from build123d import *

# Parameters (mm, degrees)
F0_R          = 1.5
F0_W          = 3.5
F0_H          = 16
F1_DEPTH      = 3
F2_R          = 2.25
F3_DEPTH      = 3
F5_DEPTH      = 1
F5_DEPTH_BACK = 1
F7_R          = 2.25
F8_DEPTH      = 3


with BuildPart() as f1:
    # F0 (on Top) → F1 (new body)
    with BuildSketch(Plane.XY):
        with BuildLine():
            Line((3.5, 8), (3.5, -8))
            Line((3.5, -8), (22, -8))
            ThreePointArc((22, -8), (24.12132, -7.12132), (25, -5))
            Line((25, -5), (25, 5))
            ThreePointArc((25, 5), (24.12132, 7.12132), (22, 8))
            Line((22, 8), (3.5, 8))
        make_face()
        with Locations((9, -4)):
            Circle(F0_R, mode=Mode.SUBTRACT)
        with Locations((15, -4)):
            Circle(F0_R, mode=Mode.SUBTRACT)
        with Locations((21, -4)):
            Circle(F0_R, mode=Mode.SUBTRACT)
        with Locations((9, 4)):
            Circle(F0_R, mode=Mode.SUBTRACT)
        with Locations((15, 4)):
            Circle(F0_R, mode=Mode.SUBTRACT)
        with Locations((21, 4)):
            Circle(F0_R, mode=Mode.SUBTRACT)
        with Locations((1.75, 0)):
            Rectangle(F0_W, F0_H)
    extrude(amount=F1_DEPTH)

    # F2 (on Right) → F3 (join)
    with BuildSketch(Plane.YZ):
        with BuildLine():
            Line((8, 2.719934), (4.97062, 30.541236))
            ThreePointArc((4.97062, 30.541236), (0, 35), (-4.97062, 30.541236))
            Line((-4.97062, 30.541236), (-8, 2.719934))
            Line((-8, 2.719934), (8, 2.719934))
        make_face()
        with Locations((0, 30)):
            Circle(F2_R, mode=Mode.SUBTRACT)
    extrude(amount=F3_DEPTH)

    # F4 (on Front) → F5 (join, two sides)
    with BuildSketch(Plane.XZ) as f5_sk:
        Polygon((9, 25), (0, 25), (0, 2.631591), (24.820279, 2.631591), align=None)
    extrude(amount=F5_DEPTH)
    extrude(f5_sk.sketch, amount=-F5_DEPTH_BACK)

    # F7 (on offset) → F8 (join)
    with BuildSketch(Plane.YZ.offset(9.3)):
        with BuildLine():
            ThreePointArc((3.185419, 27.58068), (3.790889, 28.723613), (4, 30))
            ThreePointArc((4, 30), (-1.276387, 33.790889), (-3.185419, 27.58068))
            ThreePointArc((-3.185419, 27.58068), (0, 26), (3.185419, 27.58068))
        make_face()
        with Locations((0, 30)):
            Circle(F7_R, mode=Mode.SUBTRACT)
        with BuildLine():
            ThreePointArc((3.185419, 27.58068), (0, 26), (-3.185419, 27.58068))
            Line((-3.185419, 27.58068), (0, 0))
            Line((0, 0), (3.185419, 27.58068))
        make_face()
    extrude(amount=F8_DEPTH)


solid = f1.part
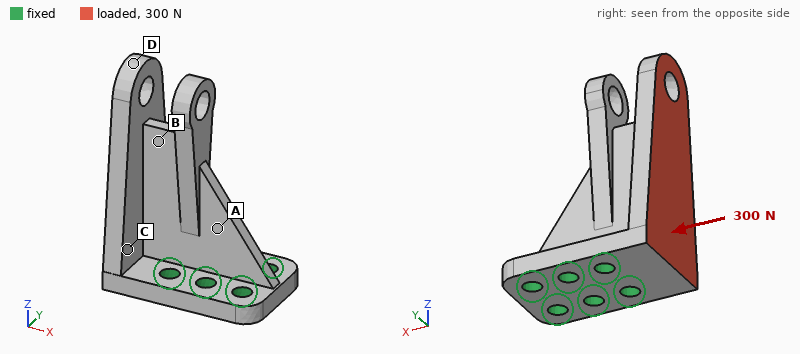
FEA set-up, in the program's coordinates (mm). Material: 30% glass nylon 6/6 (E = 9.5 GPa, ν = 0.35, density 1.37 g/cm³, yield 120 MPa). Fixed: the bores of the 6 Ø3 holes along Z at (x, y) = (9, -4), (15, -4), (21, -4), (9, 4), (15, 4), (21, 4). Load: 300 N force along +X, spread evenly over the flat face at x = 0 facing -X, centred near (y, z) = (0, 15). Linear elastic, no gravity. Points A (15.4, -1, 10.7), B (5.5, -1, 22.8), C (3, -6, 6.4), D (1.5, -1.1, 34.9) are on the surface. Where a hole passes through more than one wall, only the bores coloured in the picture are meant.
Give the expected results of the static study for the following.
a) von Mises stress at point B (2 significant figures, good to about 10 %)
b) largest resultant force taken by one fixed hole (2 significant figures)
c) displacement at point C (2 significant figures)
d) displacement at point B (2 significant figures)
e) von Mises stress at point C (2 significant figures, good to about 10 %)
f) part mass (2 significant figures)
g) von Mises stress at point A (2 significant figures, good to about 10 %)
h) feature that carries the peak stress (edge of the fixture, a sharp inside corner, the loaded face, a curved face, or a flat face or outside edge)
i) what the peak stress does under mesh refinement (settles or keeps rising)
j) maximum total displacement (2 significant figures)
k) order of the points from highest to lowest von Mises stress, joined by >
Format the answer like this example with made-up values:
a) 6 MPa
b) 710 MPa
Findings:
a) 14 MPa
b) 150 N
c) 0.041 mm
d) 0.10 mm
e) 6.9 MPa
f) 4.1 g
g) 17 MPa
h) edge of the fixture
i) keeps rising
j) 0.24 mm
k) A > B > C > D
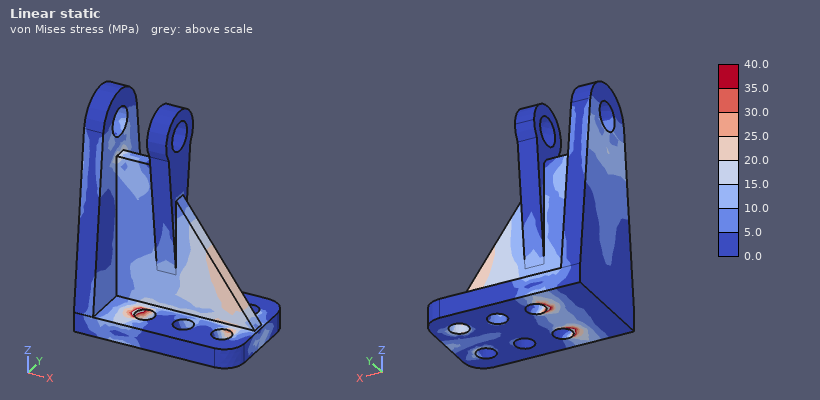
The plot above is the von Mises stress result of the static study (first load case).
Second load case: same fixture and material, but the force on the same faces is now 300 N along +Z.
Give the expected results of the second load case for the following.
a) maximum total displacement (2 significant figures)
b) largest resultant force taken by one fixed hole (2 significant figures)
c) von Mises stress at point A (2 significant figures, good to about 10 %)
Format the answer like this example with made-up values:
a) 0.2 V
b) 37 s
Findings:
a) 0.16 mm
b) 220 N
c) 9.1 MPa
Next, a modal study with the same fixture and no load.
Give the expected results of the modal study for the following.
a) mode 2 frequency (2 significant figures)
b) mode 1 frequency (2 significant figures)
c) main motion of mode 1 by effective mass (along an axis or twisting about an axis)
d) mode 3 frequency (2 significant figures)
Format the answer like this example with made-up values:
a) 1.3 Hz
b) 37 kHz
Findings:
a) 4500 Hz
b) 2300 Hz
c) along Y
d) 4600 Hz
